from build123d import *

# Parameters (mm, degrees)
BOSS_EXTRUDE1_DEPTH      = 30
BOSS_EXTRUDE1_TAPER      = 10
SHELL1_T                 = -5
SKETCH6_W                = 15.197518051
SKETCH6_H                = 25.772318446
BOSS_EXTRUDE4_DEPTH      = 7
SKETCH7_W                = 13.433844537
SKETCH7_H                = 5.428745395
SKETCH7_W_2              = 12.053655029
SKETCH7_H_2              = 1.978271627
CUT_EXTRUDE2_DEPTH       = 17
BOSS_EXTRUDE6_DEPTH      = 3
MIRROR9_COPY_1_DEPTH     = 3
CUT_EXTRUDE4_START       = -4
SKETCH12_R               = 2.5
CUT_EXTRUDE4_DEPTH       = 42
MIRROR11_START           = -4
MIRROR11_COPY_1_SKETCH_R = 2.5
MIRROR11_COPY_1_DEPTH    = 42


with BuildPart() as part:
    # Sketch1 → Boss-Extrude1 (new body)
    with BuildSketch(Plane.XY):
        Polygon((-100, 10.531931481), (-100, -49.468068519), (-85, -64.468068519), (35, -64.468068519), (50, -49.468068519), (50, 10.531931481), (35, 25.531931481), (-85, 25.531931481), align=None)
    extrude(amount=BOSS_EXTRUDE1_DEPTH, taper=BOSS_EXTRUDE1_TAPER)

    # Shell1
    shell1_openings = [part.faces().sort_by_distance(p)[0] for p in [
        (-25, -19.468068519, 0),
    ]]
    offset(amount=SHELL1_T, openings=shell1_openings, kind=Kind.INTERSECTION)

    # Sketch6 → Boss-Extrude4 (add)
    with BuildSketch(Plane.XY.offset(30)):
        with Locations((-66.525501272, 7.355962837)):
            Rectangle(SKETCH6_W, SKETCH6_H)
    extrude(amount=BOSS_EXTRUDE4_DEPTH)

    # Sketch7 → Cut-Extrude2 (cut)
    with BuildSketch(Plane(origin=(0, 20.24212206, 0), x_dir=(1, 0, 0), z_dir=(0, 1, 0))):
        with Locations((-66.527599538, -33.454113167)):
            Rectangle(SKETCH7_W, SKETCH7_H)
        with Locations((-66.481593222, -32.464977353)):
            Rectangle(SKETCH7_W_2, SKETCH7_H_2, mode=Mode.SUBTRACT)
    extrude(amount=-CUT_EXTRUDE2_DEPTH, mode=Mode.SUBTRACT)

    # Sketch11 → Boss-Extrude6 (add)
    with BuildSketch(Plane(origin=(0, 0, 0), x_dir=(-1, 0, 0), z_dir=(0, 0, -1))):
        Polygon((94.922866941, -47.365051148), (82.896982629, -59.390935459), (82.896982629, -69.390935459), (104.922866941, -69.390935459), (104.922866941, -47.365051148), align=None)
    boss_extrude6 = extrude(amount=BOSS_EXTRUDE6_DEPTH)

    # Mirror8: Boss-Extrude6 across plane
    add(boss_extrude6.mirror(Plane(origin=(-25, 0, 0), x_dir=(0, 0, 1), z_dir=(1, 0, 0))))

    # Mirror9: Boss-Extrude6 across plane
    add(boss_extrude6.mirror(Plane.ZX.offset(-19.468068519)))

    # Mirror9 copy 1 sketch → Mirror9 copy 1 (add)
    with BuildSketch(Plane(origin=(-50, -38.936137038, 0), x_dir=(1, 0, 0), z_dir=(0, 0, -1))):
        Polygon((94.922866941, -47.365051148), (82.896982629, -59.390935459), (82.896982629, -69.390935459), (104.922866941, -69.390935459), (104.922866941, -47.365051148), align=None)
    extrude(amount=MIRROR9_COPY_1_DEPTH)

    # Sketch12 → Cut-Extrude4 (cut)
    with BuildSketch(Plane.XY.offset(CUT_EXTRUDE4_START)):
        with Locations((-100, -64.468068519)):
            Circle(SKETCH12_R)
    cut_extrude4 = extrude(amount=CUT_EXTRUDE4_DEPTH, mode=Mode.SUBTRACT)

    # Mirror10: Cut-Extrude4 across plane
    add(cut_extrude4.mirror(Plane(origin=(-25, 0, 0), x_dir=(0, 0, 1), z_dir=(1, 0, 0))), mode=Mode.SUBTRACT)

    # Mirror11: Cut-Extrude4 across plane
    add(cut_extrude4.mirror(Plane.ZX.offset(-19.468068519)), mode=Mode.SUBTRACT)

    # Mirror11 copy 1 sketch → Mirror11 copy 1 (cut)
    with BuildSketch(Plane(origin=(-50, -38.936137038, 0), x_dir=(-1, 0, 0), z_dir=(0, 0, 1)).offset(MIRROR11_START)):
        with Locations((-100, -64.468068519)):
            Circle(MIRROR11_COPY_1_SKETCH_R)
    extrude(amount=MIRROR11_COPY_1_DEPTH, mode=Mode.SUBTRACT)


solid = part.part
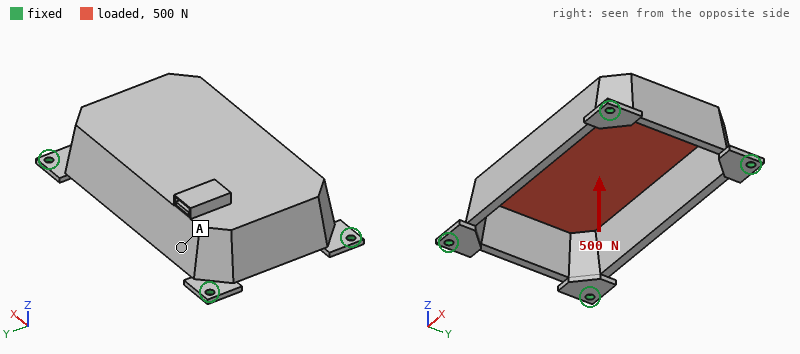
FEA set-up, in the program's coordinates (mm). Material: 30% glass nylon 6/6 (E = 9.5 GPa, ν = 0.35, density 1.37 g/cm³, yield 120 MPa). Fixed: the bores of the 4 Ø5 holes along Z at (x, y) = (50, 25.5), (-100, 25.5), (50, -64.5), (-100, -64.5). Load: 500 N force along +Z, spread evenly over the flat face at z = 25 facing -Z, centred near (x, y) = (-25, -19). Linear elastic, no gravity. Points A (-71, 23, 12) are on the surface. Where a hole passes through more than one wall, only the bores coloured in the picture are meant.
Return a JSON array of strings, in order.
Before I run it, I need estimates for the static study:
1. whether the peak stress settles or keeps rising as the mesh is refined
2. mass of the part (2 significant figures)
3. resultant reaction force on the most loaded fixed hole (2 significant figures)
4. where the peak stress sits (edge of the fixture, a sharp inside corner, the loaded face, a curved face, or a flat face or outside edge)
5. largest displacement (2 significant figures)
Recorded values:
["keeps rising", "160 g", "180 N", "edge of the fixture", "0.15 mm"]
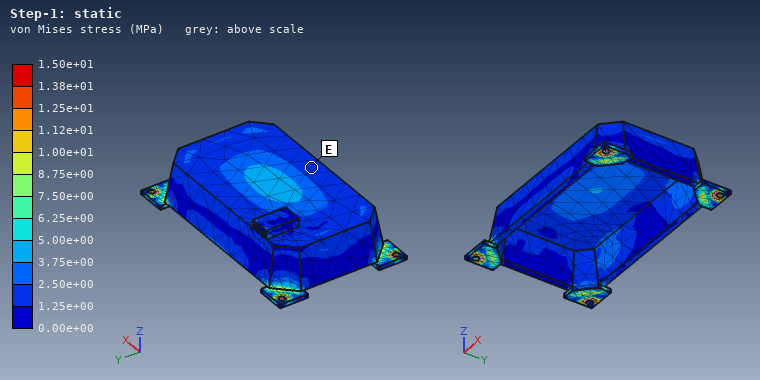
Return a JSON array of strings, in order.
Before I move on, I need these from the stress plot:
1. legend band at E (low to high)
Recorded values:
["1.25e+00 to 2.50e+00 MPa"]
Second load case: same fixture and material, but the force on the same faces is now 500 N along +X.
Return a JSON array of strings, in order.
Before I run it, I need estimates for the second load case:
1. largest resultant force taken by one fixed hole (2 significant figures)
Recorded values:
["140 N"]
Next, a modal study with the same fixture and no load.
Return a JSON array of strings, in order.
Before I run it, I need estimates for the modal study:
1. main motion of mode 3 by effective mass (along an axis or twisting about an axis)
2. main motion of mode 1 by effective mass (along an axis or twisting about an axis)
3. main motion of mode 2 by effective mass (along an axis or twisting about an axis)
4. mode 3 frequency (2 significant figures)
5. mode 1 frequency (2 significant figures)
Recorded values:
["along Y", "along Z", "along Y", "1600 Hz", "1100 Hz"]
